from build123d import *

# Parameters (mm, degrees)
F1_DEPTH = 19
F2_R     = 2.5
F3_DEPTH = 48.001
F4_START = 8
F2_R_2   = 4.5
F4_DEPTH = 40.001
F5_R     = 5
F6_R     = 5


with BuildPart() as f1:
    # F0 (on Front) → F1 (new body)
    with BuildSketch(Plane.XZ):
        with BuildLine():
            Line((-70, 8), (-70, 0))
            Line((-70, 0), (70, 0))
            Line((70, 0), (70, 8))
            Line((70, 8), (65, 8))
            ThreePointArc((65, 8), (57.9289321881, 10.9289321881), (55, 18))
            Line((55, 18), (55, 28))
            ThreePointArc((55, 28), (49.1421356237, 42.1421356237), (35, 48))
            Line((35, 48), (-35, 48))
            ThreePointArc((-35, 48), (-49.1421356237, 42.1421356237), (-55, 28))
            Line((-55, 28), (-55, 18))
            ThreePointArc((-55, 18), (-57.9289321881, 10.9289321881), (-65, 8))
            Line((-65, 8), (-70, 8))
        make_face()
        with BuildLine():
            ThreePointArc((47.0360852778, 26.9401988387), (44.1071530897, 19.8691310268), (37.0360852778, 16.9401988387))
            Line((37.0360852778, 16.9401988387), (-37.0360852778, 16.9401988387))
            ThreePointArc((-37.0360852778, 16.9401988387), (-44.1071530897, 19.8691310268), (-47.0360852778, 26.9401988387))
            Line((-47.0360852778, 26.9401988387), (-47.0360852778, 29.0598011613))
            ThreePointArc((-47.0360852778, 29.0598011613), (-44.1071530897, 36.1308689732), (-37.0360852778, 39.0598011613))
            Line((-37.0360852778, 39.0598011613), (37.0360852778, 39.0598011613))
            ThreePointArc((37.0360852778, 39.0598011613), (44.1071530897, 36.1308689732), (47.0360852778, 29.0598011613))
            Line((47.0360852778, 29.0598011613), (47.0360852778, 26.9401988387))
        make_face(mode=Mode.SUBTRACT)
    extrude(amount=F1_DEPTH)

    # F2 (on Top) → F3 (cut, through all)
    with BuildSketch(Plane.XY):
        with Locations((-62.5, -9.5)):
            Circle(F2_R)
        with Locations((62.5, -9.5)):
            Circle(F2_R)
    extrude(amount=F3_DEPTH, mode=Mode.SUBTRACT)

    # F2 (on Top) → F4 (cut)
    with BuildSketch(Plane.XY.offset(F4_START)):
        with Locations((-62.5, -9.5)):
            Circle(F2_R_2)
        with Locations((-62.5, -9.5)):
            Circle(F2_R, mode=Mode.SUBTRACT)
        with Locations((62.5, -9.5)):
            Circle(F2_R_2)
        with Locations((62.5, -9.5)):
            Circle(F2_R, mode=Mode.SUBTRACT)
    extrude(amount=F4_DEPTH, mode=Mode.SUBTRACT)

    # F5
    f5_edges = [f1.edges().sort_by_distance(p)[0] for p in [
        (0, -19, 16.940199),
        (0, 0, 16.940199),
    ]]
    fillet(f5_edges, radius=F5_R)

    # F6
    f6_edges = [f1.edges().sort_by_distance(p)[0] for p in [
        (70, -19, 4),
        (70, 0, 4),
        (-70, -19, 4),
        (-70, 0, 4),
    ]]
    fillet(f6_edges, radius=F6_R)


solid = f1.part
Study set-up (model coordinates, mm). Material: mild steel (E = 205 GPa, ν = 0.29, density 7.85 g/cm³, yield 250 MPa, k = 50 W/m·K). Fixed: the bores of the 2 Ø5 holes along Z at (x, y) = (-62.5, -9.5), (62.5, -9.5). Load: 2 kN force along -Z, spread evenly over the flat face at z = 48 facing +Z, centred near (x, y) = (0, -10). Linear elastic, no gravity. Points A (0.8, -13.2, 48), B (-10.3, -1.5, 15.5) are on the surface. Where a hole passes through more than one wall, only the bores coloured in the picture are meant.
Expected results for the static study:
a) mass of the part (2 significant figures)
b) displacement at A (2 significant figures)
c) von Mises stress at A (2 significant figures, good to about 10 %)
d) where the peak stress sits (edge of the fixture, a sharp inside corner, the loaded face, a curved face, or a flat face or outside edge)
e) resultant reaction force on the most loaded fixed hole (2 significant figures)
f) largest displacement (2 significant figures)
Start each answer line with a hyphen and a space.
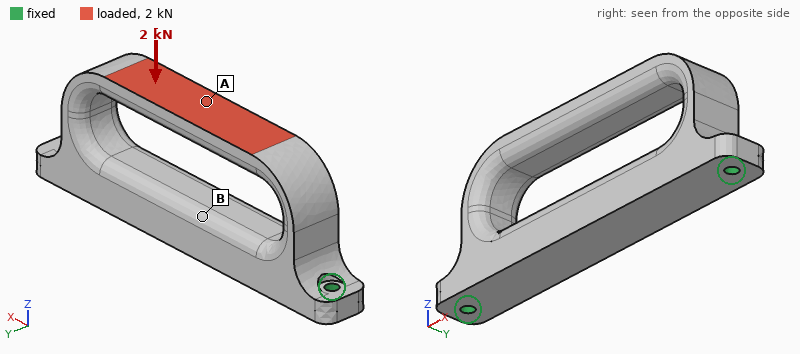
- 480 g
- 49 µm
- 63 MPa
- a curved face
- 1.1 kN
- 50 µm
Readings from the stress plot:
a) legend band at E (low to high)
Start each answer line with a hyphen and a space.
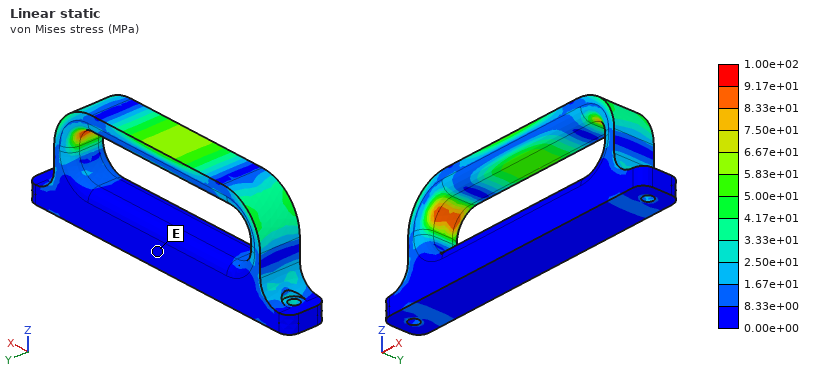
- 0.00e+00 to 8.33e+00 MPa
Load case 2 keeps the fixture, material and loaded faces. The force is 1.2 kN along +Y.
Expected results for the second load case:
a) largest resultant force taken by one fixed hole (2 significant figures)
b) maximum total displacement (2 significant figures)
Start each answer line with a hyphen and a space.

- 600 N
- 72 µm
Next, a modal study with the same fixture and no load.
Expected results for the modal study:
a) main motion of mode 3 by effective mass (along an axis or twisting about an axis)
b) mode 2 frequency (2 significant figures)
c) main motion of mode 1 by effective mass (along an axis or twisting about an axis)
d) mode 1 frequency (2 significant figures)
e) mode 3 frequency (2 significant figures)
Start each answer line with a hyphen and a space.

- along X
- 3600 Hz
- along Y
- 2100 Hz
- 3900 Hz
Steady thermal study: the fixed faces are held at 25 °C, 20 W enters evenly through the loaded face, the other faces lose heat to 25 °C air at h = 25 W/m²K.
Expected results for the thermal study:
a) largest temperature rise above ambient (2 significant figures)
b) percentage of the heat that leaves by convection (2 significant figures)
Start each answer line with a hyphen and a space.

- 67 K
- 39 %
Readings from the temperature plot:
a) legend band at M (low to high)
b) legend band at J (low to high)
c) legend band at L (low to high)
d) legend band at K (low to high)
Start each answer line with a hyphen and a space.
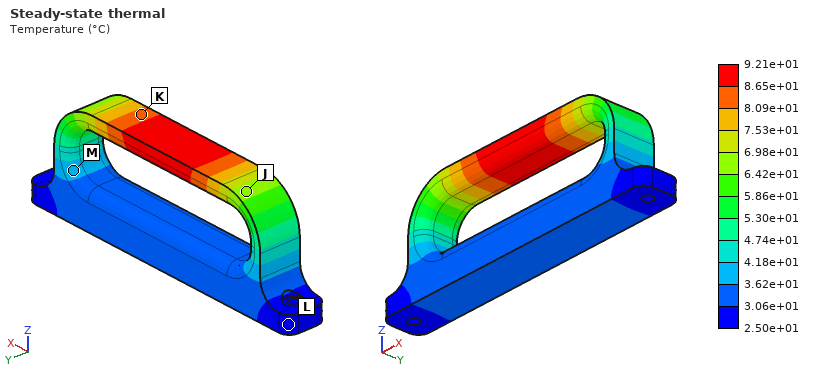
- 3.62e+01 to 4.18e+01 °C
- 6.42e+01 to 6.98e+01 °C
- 2.50e+01 to 3.06e+01 °C
- 8.09e+01 to 8.65e+01 °C
